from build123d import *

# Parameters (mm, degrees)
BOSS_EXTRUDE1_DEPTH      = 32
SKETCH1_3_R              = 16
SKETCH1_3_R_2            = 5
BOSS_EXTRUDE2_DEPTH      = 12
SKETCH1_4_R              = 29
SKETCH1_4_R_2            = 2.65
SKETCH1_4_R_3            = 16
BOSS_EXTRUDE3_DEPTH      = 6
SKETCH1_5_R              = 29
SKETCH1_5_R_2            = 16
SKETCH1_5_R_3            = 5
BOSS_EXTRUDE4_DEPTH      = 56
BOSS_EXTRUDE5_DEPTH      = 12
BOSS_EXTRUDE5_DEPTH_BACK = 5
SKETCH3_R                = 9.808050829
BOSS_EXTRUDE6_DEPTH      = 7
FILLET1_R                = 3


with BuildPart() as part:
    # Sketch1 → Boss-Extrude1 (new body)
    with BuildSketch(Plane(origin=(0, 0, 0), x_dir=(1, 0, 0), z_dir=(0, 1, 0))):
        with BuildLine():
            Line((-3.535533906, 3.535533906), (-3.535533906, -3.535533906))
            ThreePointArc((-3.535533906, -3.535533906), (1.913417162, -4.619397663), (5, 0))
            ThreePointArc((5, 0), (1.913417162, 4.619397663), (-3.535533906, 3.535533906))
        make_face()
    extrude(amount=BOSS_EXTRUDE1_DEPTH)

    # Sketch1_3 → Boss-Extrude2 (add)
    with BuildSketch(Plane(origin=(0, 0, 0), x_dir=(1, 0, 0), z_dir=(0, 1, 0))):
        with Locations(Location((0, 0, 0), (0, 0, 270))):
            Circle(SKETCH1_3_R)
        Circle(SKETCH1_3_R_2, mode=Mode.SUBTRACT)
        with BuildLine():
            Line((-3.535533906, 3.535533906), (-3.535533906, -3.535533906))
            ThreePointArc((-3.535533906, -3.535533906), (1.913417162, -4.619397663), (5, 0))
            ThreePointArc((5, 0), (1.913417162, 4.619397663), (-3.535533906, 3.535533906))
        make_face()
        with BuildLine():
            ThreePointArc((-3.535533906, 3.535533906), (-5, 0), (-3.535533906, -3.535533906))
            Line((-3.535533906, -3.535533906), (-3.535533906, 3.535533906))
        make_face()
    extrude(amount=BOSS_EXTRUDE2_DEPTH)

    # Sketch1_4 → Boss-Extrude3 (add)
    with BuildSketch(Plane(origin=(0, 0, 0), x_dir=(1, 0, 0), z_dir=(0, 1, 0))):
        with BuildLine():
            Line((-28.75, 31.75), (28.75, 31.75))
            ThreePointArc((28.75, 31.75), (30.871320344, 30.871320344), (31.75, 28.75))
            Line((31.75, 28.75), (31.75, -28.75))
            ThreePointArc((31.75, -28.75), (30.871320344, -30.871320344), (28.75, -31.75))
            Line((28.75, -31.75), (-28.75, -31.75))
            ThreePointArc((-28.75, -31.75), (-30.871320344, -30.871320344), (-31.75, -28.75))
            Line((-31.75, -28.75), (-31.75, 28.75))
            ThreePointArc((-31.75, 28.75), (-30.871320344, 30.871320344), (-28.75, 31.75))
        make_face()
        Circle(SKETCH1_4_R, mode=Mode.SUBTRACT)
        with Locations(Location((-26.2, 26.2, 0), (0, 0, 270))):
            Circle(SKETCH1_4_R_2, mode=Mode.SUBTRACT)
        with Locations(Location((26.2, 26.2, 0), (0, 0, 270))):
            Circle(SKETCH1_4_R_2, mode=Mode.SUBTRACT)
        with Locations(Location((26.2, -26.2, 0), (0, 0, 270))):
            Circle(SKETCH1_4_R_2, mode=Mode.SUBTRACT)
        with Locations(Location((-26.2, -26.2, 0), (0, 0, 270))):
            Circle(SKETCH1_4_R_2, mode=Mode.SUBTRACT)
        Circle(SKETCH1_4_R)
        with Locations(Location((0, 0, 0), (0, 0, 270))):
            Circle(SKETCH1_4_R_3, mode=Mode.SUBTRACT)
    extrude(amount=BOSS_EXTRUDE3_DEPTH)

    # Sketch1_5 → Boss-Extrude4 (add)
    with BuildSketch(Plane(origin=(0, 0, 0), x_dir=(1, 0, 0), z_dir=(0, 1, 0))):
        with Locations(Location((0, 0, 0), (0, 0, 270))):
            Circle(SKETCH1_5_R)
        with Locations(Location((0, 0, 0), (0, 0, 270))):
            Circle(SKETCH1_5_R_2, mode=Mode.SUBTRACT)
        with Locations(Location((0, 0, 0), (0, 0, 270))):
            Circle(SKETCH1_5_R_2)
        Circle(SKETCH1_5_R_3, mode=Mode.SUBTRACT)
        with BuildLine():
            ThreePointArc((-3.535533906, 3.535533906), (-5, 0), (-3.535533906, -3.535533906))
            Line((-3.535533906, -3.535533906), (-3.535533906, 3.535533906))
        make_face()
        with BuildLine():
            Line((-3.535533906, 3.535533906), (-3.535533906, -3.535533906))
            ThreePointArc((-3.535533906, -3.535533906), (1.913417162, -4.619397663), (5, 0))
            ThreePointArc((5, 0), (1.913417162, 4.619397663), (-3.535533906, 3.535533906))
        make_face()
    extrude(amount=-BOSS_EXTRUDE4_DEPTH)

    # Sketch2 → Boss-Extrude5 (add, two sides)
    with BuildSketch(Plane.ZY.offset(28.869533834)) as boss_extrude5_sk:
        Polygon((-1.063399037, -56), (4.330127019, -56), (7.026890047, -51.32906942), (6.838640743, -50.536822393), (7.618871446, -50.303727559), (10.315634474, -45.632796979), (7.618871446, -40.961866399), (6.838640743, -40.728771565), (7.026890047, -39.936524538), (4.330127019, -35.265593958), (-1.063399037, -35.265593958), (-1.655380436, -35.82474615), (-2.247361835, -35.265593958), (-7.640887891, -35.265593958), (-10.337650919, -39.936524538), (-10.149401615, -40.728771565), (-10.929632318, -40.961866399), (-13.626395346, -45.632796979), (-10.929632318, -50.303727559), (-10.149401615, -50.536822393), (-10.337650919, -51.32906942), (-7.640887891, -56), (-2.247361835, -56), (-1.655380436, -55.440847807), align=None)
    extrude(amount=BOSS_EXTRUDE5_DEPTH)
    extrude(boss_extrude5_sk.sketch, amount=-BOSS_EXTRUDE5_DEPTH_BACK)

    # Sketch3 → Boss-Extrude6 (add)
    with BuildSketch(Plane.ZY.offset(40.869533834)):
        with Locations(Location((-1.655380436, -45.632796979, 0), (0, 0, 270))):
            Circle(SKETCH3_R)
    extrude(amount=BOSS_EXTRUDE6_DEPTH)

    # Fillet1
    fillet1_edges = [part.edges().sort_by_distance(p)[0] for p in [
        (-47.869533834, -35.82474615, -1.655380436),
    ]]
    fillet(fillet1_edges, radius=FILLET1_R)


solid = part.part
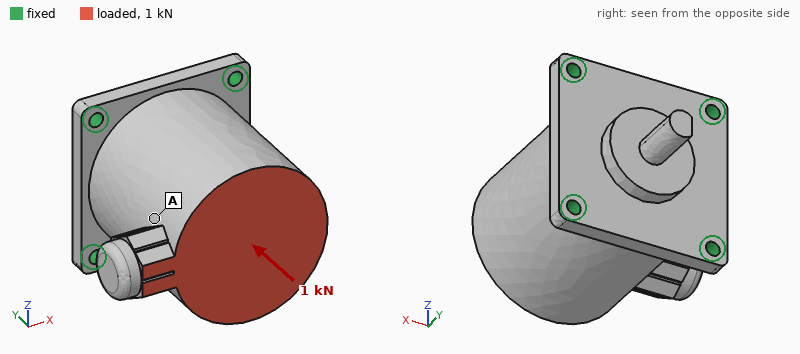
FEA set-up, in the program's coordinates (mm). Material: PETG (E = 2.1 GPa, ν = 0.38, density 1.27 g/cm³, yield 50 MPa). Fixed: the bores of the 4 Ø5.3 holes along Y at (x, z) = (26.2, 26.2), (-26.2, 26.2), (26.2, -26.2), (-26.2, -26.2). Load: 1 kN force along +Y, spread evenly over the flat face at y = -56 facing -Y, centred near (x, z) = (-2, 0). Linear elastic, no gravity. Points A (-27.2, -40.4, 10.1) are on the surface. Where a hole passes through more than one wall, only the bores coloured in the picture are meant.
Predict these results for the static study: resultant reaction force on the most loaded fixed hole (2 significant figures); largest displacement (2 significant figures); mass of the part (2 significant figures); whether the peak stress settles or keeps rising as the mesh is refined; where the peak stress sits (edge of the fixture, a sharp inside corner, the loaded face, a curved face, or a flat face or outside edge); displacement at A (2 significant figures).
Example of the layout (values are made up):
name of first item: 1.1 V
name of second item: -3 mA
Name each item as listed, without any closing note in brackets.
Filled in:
resultant reaction force on the most loaded fixed hole: 290 N
largest displacement: 97 µm
mass of the part: 230 g
whether the peak stress settles or keeps rising as the mesh is refined: keeps rising
where the peak stress sits: edge of the fixture
displacement at A: 84 µm
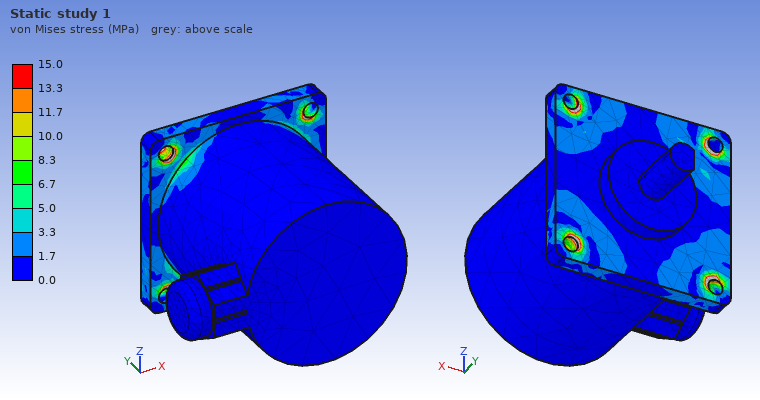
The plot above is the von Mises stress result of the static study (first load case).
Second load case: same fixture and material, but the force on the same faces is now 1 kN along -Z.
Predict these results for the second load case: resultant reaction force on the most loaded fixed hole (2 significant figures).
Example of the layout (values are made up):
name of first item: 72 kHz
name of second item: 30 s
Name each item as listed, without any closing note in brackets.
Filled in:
resultant reaction force on the most loaded fixed hole: 710 N
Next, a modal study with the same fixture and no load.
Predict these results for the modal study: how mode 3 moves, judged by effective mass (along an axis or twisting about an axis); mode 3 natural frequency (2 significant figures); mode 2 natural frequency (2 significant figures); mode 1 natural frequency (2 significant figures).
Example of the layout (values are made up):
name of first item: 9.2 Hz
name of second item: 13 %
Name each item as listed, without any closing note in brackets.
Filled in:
how mode 3 moves, judged by effective mass: along Y
mode 3 natural frequency: 1200 Hz
mode 2 natural frequency: 770 Hz
mode 1 natural frequency: 750 Hz
